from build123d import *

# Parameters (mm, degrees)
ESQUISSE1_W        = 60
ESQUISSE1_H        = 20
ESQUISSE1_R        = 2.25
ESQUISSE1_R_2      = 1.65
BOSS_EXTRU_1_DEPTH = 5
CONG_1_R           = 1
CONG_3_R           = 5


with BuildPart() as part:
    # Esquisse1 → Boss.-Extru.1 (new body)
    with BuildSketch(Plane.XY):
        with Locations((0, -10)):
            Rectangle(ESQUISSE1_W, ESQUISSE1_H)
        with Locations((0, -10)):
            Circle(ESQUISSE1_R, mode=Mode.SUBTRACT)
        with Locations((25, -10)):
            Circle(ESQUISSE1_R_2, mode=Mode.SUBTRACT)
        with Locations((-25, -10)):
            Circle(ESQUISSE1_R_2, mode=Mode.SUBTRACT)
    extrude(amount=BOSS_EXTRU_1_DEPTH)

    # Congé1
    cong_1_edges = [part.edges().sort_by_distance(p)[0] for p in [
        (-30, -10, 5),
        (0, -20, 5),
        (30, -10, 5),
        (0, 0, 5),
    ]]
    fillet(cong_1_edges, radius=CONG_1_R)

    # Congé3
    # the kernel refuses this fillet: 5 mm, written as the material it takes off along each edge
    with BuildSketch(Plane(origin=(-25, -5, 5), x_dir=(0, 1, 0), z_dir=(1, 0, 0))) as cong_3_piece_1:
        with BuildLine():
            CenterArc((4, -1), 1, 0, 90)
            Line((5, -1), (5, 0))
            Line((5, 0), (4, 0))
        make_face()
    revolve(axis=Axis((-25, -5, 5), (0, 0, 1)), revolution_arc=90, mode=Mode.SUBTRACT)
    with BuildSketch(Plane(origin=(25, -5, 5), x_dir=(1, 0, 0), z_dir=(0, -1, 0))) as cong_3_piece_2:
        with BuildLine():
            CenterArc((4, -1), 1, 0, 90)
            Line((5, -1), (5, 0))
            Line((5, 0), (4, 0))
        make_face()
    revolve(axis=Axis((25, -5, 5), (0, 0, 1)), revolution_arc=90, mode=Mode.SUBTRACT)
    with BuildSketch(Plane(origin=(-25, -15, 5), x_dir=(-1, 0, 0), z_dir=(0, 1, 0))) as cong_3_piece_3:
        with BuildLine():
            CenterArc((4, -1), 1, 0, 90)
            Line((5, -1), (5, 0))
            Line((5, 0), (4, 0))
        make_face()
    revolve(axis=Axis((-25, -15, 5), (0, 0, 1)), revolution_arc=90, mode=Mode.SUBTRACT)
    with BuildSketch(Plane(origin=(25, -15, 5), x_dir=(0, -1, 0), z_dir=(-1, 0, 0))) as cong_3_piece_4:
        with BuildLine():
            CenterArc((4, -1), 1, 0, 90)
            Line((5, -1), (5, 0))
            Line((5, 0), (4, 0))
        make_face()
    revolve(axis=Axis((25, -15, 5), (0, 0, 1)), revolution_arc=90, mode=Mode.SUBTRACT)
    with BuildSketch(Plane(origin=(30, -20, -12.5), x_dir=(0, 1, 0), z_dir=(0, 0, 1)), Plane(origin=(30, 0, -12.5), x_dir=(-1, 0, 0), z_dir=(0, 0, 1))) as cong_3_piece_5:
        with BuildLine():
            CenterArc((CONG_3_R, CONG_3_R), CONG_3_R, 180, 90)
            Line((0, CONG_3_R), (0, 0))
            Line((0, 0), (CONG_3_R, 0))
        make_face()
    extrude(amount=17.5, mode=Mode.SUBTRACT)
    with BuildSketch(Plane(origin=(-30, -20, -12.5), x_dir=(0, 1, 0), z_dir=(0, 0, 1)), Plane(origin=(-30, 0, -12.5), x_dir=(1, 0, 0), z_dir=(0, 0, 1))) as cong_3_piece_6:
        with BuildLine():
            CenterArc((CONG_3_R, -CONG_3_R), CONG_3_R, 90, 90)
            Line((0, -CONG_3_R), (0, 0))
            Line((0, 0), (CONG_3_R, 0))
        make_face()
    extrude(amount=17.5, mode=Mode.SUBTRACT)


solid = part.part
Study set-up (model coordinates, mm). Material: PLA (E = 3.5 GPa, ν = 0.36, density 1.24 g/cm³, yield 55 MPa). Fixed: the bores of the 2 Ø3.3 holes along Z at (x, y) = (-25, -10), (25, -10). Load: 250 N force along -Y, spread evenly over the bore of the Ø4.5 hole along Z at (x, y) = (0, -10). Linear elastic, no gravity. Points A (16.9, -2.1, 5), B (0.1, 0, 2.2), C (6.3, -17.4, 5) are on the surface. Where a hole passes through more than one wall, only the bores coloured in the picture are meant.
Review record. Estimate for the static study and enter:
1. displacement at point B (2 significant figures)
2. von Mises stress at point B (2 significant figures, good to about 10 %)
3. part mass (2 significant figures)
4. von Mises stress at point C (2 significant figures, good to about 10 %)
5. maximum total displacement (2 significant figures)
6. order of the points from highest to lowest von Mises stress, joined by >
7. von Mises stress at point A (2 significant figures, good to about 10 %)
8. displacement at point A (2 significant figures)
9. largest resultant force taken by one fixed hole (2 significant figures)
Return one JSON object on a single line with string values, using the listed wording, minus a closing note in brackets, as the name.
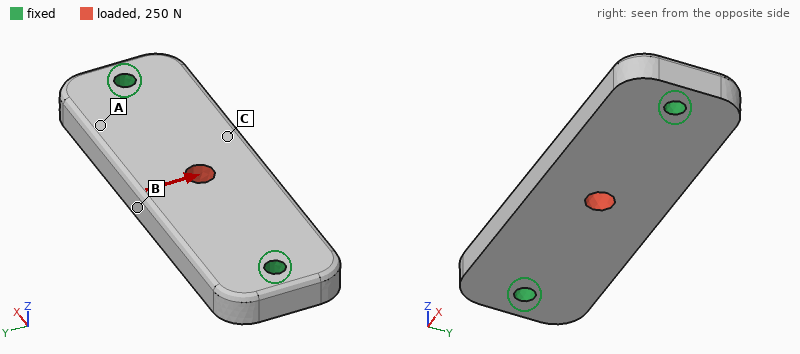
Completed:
{"displacement at point B": "64 µm", "von Mises stress at point B": "8.4 MPa", "part mass": "7.1 g", "von Mises stress at point C": "4.4 MPa", "maximum total displacement": "70 µm", "order of the points from highest to lowest von Mises stress, joined by >": "B > C > A", "von Mises stress at point A": "1.7 MPa", "displacement at point A": "32 µm", "largest resultant force taken by one fixed hole": "130 N"}
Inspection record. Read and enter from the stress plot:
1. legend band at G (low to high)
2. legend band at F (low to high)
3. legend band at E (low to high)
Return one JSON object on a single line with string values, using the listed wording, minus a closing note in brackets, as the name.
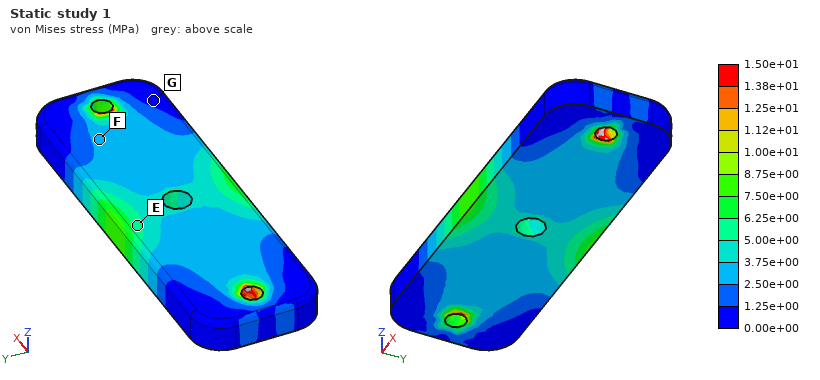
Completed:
{"legend band at G": "0.00e+00 to 1.25e+00 MPa", "legend band at F": "2.50e+00 to 3.75e+00 MPa", "legend band at E": "5.00e+00 to 6.25e+00 MPa"}
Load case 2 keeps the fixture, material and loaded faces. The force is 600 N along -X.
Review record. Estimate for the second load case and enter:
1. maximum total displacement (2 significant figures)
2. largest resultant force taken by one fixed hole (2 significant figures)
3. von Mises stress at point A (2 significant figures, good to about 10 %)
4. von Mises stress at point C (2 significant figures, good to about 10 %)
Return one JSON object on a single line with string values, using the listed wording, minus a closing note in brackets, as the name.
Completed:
{"maximum total displacement": "36 µm", "largest resultant force taken by one fixed hole": "300 N", "von Mises stress at point A": "2.1 MPa", "von Mises stress at point C": "2.0 MPa"}
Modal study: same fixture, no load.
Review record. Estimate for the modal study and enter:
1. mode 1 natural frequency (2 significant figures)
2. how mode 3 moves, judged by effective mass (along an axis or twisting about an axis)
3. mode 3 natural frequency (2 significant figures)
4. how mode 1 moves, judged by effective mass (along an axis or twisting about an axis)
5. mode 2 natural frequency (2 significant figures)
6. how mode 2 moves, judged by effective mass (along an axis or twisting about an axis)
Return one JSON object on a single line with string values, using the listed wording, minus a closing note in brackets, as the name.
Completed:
{"mode 1 natural frequency": "3000 Hz", "how mode 3 moves, judged by effective mass": "along Y", "mode 3 natural frequency": "5700 Hz", "how mode 1 moves, judged by effective mass": "along Z", "mode 2 natural frequency": "4400 Hz", "how mode 2 moves, judged by effective mass": "twisting about X"}
